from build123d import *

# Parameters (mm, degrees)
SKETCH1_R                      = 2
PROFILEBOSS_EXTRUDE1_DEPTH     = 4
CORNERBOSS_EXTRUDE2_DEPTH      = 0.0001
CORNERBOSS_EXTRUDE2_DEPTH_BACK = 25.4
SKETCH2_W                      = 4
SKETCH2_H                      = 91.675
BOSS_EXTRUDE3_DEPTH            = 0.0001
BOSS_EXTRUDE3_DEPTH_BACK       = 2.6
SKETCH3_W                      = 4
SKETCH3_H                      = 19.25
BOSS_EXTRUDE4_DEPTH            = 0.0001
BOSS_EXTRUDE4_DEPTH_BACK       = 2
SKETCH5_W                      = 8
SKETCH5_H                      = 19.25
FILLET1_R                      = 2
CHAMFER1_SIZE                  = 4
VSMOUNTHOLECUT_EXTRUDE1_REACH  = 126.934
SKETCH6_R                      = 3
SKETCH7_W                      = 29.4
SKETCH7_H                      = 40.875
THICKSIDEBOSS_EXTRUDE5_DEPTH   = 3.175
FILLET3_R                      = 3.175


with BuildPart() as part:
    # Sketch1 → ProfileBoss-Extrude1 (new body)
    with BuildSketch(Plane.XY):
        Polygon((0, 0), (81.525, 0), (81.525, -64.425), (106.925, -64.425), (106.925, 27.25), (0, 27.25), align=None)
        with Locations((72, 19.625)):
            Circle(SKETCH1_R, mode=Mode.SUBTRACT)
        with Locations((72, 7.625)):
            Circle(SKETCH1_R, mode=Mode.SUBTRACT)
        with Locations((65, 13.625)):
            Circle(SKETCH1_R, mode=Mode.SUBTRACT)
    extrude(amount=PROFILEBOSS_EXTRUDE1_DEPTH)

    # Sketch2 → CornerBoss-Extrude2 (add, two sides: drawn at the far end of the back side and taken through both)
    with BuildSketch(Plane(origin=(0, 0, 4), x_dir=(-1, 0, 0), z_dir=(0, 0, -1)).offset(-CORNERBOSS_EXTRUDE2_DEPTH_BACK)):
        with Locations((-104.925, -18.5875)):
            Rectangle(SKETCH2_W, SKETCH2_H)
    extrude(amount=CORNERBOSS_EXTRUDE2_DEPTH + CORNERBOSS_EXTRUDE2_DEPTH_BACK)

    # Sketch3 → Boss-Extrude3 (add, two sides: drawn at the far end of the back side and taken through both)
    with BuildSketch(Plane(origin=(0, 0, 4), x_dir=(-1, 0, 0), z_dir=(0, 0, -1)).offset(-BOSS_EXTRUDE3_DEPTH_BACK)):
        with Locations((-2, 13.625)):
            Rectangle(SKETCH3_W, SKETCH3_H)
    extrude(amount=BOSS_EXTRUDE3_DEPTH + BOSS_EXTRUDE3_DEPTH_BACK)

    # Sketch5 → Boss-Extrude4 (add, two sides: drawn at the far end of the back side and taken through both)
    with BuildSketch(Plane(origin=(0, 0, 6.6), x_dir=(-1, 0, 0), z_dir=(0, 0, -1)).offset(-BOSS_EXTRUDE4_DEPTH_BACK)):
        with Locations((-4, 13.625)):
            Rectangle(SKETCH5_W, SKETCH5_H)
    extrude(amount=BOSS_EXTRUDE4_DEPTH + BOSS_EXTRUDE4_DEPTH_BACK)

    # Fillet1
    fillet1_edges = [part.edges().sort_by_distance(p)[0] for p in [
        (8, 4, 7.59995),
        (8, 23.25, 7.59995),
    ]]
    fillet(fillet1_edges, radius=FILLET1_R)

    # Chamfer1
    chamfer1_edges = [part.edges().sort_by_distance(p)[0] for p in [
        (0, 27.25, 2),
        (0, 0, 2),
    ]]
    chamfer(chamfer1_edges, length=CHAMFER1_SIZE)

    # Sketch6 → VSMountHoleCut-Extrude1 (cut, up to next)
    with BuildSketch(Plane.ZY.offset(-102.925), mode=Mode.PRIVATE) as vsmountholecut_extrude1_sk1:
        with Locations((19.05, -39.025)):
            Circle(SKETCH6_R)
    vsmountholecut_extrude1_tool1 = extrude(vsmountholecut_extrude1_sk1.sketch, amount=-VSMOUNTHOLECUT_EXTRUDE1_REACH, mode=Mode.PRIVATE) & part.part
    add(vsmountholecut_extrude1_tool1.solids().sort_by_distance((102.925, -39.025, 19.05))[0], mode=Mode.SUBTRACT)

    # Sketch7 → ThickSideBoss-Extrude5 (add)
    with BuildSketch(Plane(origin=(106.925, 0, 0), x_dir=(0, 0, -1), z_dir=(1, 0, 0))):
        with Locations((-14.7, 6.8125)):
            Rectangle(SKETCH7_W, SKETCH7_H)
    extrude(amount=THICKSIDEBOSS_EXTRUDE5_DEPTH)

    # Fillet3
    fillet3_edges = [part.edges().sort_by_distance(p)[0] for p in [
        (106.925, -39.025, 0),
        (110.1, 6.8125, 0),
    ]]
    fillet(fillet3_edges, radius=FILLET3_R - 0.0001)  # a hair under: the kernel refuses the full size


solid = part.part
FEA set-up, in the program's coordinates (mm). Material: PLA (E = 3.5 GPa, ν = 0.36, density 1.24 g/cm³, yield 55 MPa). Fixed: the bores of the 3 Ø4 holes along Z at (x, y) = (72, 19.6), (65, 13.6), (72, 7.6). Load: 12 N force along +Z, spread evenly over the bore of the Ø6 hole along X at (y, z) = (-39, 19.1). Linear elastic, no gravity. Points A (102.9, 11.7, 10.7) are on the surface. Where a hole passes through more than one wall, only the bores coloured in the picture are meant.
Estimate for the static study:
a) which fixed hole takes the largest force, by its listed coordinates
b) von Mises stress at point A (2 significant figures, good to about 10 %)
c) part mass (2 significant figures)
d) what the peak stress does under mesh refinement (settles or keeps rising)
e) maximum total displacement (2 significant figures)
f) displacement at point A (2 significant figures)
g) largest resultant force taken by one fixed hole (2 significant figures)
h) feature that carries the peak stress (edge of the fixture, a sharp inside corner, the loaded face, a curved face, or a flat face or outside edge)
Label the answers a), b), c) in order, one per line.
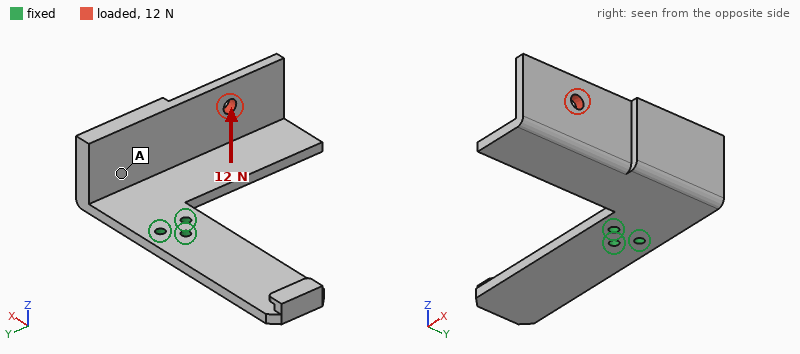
a) (72, 7.6)
b) 1.0 MPa
c) 39 g
d) keeps rising
e) 1.6 mm
f) 0.29 mm
g) 46 N
h) edge of the fixture
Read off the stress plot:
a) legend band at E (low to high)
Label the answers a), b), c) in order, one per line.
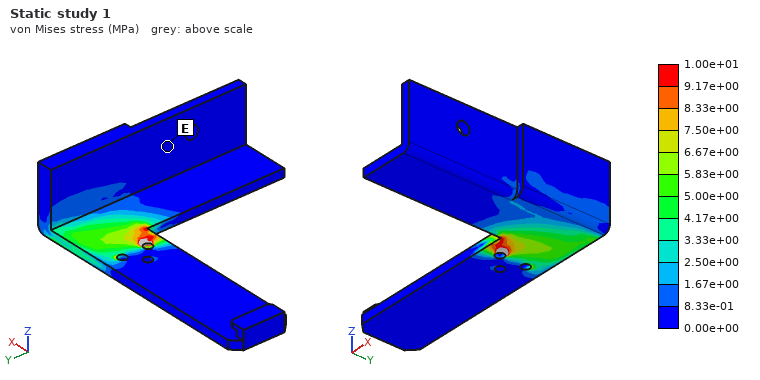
a) 0.00e+00 to 8.33e-01 MPa
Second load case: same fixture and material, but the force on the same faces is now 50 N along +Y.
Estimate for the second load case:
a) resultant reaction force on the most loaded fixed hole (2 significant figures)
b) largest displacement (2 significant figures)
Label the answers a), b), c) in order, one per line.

a) 110 N
b) 1.7 mm
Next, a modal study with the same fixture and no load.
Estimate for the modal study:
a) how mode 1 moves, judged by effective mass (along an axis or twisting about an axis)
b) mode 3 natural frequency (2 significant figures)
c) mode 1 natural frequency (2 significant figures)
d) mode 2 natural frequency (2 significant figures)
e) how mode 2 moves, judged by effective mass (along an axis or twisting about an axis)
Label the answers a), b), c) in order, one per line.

a) along Z
b) 270 Hz
c) 140 Hz
d) 240 Hz
e) along Z
